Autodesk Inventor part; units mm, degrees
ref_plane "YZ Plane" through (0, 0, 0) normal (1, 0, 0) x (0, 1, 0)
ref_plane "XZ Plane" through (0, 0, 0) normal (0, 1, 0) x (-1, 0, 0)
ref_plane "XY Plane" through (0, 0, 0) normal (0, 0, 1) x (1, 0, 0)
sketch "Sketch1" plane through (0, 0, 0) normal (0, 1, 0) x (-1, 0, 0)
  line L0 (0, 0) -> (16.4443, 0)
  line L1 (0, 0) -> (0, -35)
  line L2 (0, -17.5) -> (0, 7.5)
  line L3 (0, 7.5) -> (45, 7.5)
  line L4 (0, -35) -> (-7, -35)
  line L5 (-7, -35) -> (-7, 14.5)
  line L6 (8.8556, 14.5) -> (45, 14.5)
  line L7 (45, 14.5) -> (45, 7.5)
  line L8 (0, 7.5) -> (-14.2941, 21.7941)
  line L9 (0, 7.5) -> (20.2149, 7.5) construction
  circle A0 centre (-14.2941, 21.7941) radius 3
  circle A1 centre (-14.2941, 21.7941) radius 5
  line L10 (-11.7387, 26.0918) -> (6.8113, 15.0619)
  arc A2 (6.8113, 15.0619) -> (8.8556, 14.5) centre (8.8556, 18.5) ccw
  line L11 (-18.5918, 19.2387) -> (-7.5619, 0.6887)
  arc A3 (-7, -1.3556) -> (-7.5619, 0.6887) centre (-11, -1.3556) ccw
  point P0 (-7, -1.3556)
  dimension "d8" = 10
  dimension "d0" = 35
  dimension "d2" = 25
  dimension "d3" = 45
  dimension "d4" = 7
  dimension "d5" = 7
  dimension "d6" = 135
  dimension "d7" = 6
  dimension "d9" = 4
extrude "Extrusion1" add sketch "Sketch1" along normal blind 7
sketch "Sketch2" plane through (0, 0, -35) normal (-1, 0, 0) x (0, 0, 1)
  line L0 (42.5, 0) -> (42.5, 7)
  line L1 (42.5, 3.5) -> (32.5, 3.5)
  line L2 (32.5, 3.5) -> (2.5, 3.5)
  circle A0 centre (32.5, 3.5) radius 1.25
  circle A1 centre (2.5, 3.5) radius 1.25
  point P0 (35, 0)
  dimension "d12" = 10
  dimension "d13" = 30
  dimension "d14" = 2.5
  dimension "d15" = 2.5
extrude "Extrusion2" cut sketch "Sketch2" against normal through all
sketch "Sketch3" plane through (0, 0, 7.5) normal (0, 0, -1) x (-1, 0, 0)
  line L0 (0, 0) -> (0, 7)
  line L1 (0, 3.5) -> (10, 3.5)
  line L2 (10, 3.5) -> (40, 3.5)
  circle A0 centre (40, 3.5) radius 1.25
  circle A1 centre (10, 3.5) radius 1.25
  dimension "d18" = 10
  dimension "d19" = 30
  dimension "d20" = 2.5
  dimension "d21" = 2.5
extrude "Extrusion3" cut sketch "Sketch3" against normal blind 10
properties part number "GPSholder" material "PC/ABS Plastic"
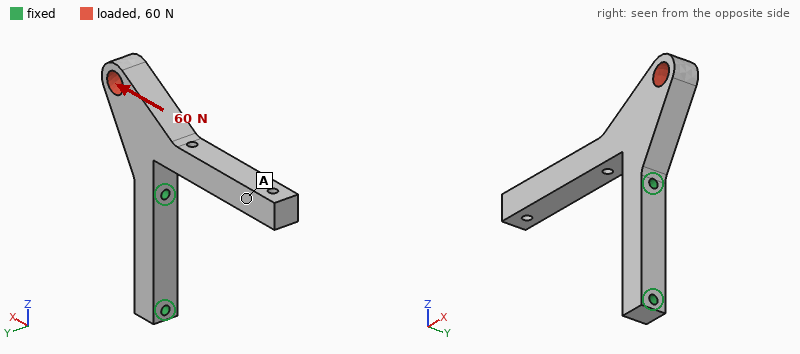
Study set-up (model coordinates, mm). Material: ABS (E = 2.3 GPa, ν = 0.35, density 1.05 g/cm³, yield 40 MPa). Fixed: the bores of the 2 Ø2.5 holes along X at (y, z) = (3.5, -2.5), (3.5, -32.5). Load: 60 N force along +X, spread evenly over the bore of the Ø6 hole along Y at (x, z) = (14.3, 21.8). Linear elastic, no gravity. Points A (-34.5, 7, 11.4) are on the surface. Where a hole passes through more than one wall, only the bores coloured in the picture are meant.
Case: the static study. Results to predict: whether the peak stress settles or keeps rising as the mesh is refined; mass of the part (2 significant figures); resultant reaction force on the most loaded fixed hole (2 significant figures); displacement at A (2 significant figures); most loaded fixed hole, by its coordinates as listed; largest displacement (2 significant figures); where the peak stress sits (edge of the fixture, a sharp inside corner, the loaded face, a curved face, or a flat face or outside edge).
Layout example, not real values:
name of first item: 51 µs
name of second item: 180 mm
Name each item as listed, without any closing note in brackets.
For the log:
whether the peak stress settles or keeps rising as the mesh is refined: keeps rising
mass of the part: 6.4 g
resultant reaction force on the most loaded fixed hole: 64 N
displacement at A: 0.78 mm
most loaded fixed hole, by its coordinates as listed: (3.5, -2.5)
largest displacement: 1.0 mm
where the peak stress sits: edge of the fixture
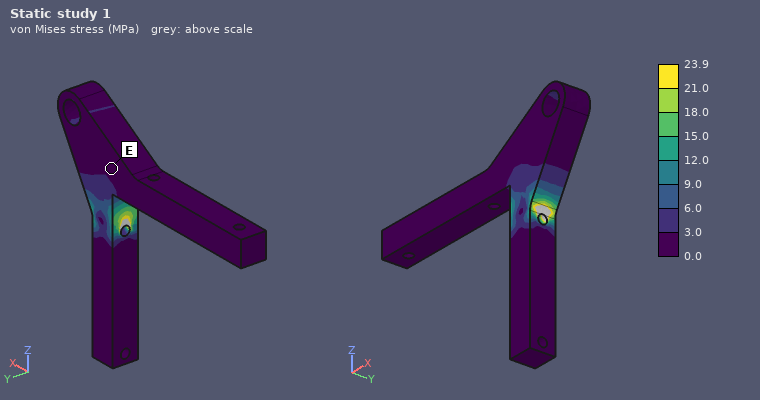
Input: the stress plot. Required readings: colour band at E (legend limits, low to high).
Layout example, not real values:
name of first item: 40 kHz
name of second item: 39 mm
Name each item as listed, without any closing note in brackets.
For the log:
colour band at E: 0.0 to 3.0 MPa
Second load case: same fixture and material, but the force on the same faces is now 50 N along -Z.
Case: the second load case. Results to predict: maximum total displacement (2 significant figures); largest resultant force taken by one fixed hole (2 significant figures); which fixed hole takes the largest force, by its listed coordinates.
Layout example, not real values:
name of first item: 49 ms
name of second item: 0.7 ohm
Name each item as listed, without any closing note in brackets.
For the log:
maximum total displacement: 0.41 mm
largest resultant force taken by one fixed hole: 49 N
which fixed hole takes the largest force, by its listed coordinates: (3.5, -2.5)
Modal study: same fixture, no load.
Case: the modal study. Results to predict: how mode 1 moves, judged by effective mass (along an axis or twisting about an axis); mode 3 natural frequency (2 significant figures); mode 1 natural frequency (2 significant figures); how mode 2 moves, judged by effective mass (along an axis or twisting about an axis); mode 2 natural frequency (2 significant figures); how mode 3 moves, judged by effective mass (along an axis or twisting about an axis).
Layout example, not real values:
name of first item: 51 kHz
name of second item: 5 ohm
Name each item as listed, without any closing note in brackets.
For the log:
how mode 1 moves, judged by effective mass: along Y
mode 3 natural frequency: 1300 Hz
mode 1 natural frequency: 500 Hz
how mode 2 moves, judged by effective mass: along Z
mode 2 natural frequency: 600 Hz
how mode 3 moves, judged by effective mass: along Y
